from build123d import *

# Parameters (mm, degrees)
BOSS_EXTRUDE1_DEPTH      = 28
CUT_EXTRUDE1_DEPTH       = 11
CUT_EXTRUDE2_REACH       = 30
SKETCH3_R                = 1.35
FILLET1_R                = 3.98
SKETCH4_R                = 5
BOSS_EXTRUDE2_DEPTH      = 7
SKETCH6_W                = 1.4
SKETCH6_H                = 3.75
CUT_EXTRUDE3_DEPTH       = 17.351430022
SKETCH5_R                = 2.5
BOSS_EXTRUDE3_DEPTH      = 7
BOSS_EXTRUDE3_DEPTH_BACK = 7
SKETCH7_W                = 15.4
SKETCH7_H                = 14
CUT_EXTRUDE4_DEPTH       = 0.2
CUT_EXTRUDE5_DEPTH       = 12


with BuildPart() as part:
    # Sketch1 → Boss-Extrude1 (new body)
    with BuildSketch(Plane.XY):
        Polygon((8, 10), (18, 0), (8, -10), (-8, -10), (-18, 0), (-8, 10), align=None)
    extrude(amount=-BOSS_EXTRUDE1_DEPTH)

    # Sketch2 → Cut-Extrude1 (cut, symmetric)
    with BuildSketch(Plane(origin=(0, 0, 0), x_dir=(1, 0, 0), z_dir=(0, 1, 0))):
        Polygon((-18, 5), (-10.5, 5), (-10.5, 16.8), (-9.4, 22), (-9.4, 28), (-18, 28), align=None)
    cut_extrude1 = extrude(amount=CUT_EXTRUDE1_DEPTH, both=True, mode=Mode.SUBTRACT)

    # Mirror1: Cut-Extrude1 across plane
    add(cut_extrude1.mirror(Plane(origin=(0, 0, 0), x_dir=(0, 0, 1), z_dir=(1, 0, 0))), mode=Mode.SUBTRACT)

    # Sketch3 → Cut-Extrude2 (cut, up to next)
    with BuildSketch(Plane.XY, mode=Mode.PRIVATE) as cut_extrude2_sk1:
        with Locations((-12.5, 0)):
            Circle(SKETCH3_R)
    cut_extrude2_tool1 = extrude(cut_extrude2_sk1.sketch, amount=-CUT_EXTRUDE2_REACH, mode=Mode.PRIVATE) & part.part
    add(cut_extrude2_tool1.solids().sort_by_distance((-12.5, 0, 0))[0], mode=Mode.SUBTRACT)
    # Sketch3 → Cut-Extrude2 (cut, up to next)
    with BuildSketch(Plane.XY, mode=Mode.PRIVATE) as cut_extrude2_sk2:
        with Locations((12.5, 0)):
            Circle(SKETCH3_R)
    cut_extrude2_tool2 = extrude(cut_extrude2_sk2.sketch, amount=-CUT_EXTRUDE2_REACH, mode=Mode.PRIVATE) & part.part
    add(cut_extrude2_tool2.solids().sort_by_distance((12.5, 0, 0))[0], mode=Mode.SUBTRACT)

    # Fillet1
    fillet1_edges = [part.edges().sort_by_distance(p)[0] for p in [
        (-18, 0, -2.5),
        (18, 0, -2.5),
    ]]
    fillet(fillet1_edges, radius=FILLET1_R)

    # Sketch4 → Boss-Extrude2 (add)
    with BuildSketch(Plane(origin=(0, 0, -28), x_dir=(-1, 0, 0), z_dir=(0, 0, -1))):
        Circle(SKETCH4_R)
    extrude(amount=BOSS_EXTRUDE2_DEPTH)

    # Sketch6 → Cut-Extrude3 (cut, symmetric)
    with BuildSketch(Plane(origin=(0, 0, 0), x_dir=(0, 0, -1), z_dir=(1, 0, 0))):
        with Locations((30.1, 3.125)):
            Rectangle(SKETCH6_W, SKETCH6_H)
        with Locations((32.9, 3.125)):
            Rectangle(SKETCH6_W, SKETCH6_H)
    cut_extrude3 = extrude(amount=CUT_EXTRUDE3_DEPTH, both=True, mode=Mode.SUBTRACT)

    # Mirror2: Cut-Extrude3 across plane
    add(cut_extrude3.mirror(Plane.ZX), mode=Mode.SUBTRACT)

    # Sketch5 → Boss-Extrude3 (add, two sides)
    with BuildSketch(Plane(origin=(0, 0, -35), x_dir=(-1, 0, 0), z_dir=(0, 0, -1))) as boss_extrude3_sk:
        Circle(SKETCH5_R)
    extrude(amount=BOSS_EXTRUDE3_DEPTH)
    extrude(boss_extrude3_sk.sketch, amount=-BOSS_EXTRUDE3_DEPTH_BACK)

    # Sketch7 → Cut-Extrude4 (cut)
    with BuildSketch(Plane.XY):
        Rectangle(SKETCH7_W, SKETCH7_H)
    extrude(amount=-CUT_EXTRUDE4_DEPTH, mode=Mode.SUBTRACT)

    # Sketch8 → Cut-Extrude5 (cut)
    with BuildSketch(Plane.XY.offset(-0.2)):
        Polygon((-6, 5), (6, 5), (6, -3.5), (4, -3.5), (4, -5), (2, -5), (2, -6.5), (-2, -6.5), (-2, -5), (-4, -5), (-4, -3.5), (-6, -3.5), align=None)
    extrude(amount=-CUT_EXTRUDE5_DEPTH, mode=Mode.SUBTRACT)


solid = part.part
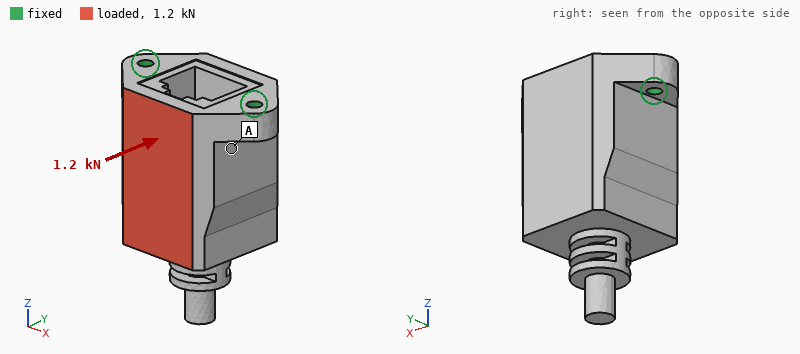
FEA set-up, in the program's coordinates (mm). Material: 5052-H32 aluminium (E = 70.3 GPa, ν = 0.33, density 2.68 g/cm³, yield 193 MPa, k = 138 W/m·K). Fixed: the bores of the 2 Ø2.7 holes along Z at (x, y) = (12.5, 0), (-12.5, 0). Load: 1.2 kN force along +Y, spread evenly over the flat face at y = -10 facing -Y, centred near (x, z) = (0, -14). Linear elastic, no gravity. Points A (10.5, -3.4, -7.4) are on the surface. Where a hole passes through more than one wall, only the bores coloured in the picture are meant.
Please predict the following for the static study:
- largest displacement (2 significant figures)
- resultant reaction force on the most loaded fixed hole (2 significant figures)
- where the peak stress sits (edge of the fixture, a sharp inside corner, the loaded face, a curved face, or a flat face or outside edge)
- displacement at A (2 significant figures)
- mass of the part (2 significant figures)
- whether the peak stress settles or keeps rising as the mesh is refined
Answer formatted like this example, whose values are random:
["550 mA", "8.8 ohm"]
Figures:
["0.11 mm", "600 N", "edge of the fixture", "0.017 mm", "29 g", "keeps rising"]
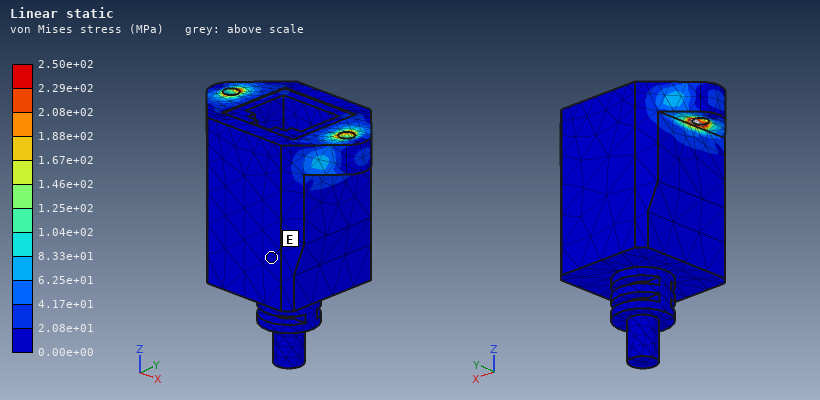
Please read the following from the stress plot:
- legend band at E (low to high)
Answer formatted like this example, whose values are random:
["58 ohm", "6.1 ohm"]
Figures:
["0.00e+00 to 2.08e+01 MPa"]
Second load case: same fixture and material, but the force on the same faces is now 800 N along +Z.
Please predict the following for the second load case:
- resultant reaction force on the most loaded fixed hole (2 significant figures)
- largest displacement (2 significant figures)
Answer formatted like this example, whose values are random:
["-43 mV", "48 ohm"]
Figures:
["430 N", "64 µm"]
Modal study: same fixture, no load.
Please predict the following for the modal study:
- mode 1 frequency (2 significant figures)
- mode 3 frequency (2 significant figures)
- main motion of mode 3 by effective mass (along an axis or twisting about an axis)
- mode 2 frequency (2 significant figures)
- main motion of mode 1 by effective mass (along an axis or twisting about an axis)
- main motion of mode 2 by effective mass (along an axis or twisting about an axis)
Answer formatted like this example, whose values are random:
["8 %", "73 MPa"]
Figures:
["3900 Hz", "18 kHz", "along Z", "11 kHz", "along Y", "along X"]
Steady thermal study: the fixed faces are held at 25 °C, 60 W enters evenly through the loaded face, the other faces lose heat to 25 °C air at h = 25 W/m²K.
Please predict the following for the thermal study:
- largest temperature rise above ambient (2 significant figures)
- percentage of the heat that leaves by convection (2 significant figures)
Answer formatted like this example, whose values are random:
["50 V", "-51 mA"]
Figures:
["39 K", "3.8 %"]
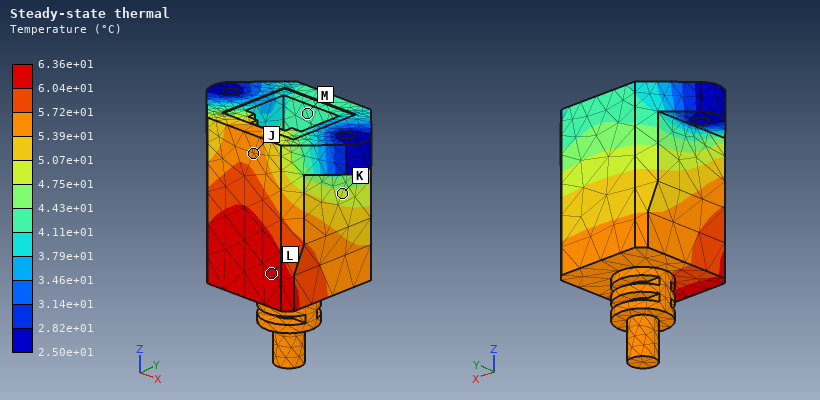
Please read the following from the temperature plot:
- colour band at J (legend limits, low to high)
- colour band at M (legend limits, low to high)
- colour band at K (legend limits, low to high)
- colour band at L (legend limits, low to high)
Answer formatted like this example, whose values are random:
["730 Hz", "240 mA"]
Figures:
["5.39e+01 to 5.72e+01 °C", "4.11e+01 to 4.43e+01 °C", "4.75e+01 to 5.07e+01 °C", "6.04e+01 to 6.36e+01 °C"]
